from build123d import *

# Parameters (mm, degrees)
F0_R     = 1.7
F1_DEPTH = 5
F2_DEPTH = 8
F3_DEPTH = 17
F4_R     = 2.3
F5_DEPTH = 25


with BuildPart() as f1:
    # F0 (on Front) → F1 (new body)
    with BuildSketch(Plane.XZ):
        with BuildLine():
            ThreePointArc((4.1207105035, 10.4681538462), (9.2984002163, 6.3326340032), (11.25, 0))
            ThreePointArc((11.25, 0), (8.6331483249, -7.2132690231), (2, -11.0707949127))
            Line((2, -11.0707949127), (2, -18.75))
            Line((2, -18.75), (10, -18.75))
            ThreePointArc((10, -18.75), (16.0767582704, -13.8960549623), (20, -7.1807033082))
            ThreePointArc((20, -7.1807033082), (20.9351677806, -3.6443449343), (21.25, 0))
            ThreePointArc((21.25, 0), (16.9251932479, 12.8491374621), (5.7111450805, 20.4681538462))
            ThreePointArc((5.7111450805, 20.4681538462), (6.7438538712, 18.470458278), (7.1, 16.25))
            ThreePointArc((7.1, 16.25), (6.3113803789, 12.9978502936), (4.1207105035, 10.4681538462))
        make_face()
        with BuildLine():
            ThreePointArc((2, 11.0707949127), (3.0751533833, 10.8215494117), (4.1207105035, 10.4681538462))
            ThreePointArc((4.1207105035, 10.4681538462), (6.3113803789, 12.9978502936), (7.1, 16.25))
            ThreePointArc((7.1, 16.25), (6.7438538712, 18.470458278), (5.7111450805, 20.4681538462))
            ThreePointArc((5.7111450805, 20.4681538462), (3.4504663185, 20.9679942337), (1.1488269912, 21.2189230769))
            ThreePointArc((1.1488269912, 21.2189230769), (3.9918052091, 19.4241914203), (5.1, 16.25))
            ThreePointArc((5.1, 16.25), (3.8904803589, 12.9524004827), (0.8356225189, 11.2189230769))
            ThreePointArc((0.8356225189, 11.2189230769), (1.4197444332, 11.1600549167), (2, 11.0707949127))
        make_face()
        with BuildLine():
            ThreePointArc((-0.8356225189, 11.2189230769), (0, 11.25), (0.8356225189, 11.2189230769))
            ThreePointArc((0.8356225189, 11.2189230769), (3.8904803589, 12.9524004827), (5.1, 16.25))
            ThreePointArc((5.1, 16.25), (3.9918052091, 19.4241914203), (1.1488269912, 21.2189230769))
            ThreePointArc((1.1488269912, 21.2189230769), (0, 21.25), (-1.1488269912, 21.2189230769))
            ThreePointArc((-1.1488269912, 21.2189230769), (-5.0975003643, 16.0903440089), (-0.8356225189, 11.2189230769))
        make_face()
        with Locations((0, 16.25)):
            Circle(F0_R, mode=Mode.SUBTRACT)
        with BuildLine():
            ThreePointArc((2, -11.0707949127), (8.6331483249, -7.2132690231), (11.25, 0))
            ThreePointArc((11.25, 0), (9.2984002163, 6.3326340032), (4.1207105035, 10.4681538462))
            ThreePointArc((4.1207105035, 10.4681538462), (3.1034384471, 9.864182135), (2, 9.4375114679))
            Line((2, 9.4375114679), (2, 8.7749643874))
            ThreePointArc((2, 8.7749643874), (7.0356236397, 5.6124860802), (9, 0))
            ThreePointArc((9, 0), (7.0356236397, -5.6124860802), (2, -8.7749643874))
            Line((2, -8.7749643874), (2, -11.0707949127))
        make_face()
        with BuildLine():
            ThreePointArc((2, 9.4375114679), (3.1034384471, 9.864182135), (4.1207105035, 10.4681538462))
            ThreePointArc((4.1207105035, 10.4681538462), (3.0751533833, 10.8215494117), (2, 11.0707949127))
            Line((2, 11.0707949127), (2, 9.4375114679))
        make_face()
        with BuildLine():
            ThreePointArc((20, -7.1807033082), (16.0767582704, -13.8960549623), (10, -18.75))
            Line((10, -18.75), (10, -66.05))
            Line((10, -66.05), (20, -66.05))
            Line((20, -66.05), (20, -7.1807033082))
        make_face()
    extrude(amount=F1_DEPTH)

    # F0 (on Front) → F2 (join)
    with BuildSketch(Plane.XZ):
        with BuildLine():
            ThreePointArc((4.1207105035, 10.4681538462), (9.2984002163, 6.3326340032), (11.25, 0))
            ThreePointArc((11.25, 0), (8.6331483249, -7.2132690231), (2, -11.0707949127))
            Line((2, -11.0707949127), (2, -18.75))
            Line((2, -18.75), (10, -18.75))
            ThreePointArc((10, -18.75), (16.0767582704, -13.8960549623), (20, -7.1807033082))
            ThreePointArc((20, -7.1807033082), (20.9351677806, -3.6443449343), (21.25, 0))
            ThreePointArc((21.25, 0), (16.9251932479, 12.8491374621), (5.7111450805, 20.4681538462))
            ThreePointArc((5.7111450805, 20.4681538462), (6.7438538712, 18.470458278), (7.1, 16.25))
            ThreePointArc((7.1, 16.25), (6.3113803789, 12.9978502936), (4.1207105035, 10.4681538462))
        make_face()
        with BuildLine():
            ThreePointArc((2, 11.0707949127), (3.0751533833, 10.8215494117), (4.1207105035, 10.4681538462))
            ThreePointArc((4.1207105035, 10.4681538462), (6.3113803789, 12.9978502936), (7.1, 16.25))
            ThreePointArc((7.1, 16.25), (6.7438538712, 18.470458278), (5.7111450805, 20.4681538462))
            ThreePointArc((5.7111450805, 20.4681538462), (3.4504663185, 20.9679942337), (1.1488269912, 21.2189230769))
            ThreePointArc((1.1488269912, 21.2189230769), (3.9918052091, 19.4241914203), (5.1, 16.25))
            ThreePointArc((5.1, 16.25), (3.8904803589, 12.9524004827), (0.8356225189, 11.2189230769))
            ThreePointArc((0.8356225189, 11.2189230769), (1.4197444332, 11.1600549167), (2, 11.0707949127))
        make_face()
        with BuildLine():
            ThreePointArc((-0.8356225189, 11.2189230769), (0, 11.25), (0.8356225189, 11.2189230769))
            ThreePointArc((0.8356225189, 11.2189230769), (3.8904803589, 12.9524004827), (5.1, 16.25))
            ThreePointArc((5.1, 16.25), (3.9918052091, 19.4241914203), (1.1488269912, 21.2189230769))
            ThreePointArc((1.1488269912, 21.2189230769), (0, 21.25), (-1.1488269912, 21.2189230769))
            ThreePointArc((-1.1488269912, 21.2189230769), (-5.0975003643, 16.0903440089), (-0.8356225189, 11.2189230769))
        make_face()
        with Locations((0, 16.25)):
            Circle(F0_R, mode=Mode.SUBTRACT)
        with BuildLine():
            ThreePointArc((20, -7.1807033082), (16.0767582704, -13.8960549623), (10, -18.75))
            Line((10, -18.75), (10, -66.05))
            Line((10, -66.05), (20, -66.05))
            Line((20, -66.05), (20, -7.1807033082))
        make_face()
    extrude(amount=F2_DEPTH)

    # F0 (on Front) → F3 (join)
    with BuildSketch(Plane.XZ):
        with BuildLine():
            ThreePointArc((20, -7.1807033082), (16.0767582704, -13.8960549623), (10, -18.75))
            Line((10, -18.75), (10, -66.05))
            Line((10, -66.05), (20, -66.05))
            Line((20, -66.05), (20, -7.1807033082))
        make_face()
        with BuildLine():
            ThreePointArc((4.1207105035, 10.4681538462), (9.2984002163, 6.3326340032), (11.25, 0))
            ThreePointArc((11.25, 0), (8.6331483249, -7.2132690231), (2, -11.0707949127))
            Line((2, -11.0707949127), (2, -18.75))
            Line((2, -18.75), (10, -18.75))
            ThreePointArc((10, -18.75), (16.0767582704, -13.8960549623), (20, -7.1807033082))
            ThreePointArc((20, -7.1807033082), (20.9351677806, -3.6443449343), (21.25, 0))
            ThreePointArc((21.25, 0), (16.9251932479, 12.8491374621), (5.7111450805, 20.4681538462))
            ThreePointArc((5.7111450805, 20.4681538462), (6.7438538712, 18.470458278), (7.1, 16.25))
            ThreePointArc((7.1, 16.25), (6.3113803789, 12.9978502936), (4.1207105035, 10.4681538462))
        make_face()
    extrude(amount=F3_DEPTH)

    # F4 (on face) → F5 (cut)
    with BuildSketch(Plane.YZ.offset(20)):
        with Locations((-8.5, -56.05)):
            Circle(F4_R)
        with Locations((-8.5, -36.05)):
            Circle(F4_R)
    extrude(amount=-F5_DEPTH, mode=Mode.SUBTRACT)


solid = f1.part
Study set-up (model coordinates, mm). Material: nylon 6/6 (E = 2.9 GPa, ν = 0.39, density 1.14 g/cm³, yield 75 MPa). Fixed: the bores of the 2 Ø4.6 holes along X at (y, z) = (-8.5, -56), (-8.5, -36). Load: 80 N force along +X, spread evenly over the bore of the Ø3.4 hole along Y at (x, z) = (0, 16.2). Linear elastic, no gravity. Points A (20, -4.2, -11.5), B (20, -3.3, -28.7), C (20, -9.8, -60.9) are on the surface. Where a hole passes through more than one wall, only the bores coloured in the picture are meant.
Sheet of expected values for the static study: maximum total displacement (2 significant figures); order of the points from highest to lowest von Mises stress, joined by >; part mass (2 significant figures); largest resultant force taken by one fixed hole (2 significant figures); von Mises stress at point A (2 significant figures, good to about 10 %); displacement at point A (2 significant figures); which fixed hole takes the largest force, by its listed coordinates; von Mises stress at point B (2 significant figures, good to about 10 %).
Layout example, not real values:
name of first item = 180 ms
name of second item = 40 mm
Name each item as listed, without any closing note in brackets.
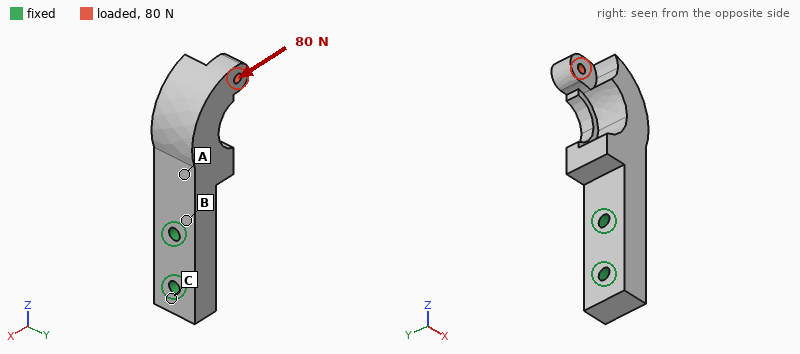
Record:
maximum total displacement = 1.1 mm
order of the points from highest to lowest von Mises stress, joined by > = B > A > C
part mass = 19 g
largest resultant force taken by one fixed hole = 120 N
von Mises stress at point A = 5.6 MPa
displacement at point A = 0.29 mm
which fixed hole takes the largest force, by its listed coordinates = (-8.5, -36)
von Mises stress at point B = 12 MPa
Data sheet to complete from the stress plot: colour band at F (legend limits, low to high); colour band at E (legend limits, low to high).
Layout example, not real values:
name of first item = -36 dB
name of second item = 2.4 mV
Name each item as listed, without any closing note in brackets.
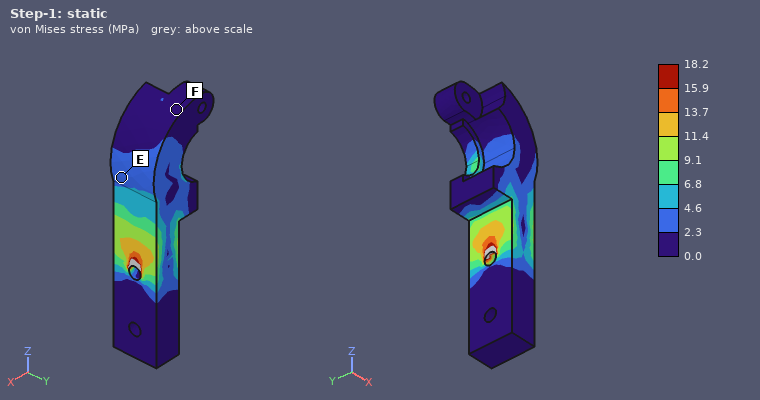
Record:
colour band at F = 0.0 to 2.3 MPa
colour band at E = 2.3 to 4.6 MPa
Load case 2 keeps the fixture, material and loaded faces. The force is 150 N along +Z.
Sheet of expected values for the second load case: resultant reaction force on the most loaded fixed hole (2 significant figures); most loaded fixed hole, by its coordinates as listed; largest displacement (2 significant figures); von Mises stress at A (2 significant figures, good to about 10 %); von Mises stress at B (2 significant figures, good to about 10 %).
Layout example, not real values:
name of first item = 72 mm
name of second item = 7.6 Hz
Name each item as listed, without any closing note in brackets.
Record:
resultant reaction force on the most loaded fixed hole = 140 N
most loaded fixed hole, by its coordinates as listed = (-8.5, -36)
largest displacement = 0.88 mm
von Mises stress at A = 3.9 MPa
von Mises stress at B = 5.8 MPa
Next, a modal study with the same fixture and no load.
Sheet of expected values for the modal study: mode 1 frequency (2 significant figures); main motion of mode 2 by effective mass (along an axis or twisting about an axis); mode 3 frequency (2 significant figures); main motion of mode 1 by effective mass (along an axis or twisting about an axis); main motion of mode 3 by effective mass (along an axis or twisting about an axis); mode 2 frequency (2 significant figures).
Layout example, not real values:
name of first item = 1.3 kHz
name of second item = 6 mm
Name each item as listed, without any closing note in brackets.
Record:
mode 1 frequency = 730 Hz
main motion of mode 2 by effective mass = along Y
mode 3 frequency = 2600 Hz
main motion of mode 1 by effective mass = along X
main motion of mode 3 by effective mass = twisting about Z
mode 2 frequency = 980 Hz
